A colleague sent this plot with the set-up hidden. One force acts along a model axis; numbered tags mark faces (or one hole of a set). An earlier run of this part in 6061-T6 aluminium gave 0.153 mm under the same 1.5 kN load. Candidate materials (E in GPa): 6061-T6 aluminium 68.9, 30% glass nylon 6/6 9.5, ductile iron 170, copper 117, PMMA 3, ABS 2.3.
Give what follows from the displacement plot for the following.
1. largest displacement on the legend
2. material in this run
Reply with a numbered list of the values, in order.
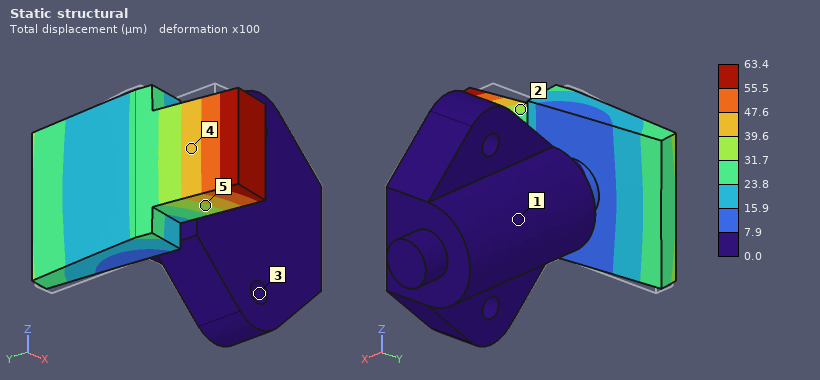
1. 63.4 µm
2. ductile iron
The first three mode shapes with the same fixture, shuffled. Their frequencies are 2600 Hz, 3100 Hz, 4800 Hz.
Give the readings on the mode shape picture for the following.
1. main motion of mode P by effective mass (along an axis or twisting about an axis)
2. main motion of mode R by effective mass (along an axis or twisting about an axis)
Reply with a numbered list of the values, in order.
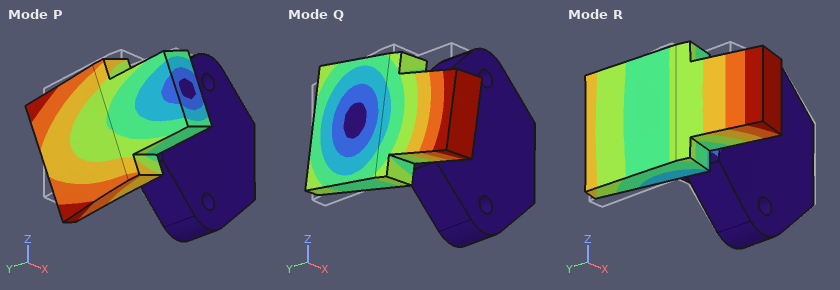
1. along Z
2. along Y
